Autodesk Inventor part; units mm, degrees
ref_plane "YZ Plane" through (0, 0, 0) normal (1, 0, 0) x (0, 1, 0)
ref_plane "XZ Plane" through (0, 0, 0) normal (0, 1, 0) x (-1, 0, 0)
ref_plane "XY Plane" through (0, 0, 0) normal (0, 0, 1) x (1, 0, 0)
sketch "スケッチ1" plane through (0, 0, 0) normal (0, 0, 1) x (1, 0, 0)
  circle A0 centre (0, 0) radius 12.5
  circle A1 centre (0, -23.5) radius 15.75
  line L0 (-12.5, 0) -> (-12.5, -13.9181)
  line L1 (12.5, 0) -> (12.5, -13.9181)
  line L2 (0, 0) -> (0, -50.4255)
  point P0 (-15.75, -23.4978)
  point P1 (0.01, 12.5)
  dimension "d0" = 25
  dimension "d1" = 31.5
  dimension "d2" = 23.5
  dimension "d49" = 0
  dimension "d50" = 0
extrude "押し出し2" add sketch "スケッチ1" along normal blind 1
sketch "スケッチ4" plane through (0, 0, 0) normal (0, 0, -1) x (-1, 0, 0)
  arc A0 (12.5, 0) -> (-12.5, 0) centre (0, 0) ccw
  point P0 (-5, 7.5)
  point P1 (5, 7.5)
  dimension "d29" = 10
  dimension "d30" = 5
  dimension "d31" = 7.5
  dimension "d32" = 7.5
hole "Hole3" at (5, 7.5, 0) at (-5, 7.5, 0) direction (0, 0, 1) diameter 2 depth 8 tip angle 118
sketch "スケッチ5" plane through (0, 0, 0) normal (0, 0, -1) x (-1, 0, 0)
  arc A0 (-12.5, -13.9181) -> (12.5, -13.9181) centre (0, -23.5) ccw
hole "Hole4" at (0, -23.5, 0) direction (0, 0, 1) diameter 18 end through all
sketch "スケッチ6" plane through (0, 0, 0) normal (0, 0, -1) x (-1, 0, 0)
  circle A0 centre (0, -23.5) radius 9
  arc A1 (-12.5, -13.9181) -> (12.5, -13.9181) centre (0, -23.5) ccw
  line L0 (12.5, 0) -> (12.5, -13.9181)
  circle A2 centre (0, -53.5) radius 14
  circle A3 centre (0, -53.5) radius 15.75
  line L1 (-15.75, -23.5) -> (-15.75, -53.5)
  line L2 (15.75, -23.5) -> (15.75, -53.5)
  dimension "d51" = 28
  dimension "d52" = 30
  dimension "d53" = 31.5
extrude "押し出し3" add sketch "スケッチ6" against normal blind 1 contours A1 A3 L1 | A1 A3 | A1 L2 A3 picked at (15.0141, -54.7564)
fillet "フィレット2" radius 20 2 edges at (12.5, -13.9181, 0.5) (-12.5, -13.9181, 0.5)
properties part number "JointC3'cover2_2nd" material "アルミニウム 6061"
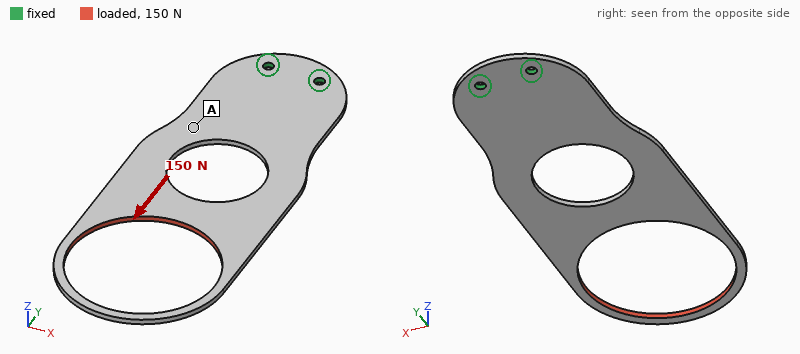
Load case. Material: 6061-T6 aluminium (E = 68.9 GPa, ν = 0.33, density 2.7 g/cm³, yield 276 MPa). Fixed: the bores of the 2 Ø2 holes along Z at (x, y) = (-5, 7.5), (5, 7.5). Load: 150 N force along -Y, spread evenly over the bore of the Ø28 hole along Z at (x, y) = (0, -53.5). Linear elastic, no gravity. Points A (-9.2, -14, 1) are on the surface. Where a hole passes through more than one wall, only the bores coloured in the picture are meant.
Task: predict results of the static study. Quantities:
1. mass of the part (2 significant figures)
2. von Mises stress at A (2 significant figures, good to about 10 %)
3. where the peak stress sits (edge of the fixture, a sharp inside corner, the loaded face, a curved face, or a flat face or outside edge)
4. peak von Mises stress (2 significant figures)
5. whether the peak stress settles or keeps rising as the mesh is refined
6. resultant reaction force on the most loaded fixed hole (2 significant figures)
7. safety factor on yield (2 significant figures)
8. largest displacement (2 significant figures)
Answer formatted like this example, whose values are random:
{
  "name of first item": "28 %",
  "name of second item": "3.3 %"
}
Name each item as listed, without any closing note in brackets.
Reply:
{
  "mass of the part": "3.6 g",
  "von Mises stress at A": "10 MPa",
  "where the peak stress sits": "the loaded face",
  "peak von Mises stress": "93 MPa",
  "whether the peak stress settles or keeps rising as the mesh is refined": "settles",
  "resultant reaction force on the most loaded fixed hole": "75 N",
  "safety factor on yield": "3.0",
  "largest displacement": "81 µm"
}
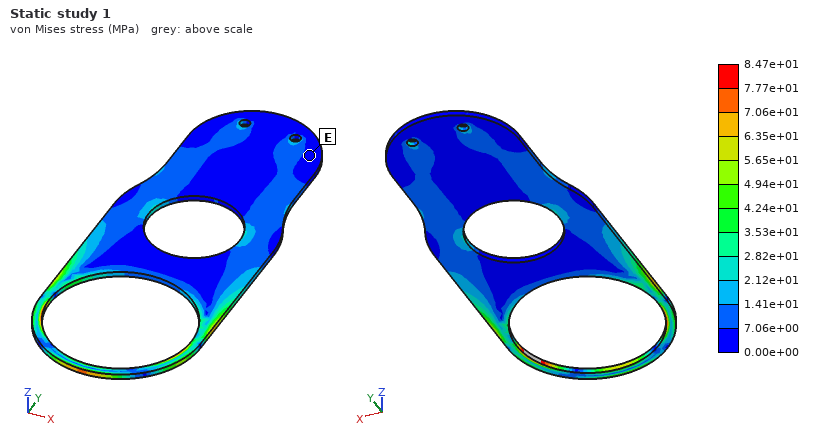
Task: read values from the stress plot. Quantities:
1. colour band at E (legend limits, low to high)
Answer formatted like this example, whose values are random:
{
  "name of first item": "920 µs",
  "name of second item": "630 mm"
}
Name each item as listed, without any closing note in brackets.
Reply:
{
  "colour band at E": "0.00e+00 to 7.06e+00 MPa"
}
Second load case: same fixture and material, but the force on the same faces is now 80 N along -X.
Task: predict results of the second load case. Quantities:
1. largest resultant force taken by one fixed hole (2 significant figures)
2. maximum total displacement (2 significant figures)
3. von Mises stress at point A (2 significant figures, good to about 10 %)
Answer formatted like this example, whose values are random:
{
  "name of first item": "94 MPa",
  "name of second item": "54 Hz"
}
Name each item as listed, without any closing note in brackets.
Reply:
{
  "largest resultant force taken by one fixed hole": "430 N",
  "maximum total displacement": "0.44 mm",
  "von Mises stress at point A": "15 MPa"
}
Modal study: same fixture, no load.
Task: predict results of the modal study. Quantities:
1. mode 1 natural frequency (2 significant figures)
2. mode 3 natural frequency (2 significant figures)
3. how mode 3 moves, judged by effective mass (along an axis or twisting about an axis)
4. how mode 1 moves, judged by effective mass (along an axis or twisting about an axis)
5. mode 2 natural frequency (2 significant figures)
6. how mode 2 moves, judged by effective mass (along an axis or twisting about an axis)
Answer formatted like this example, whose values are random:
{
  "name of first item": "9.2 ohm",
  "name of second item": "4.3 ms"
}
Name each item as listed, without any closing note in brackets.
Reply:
{
  "mode 1 natural frequency": "220 Hz",
  "mode 3 natural frequency": "880 Hz",
  "how mode 3 moves, judged by effective mass": "along Z",
  "how mode 1 moves, judged by effective mass": "along Z",
  "mode 2 natural frequency": "730 Hz",
  "how mode 2 moves, judged by effective mass": "twisting about Y"
}
